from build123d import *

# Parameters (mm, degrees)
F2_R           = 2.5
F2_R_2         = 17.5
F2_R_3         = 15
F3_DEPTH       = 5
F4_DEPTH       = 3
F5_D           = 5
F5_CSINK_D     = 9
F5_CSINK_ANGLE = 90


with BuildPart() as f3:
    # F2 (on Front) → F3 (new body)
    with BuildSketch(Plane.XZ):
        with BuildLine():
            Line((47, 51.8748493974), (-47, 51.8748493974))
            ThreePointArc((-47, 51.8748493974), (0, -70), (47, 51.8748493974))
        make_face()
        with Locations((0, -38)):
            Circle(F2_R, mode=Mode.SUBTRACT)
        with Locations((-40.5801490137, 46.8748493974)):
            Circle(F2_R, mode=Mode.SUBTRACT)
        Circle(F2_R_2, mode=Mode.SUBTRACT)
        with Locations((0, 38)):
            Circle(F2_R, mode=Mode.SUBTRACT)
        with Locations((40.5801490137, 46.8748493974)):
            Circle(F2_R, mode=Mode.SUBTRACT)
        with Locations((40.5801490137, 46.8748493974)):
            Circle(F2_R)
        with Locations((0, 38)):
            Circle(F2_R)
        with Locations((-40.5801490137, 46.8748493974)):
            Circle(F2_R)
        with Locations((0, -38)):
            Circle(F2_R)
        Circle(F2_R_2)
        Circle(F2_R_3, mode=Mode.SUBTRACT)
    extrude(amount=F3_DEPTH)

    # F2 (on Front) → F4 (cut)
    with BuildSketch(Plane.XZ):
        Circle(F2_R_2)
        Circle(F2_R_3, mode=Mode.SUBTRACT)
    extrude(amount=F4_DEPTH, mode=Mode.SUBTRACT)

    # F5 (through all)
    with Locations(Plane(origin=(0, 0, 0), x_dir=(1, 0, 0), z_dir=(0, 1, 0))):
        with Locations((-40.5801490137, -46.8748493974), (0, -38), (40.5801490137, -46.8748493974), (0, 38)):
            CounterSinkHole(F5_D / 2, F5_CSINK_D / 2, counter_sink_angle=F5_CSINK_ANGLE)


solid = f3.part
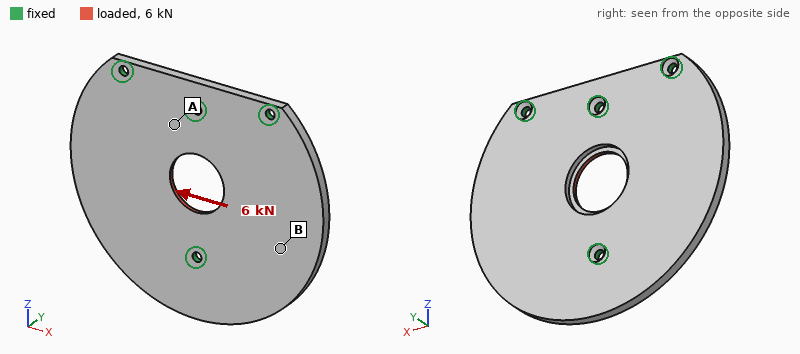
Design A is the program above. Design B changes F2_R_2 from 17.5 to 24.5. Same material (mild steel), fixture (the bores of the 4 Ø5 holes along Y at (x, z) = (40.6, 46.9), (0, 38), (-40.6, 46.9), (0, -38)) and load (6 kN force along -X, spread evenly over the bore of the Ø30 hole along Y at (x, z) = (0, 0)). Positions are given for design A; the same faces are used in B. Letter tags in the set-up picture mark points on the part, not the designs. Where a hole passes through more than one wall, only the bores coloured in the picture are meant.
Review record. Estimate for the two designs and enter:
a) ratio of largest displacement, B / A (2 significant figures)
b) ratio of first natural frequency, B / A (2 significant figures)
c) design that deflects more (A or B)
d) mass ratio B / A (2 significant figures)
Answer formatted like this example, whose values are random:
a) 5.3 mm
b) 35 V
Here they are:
a) 1.2
b) 0.99
c) B
d) 0.96
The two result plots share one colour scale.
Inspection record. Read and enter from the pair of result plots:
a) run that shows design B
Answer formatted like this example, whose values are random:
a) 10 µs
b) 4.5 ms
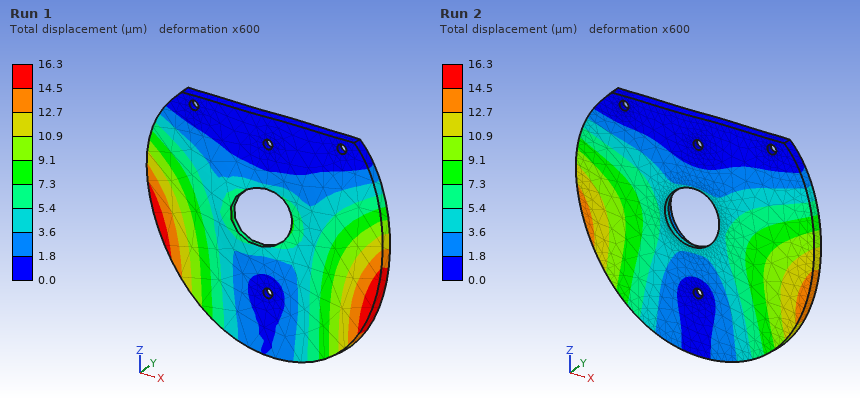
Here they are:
a) Run 1
